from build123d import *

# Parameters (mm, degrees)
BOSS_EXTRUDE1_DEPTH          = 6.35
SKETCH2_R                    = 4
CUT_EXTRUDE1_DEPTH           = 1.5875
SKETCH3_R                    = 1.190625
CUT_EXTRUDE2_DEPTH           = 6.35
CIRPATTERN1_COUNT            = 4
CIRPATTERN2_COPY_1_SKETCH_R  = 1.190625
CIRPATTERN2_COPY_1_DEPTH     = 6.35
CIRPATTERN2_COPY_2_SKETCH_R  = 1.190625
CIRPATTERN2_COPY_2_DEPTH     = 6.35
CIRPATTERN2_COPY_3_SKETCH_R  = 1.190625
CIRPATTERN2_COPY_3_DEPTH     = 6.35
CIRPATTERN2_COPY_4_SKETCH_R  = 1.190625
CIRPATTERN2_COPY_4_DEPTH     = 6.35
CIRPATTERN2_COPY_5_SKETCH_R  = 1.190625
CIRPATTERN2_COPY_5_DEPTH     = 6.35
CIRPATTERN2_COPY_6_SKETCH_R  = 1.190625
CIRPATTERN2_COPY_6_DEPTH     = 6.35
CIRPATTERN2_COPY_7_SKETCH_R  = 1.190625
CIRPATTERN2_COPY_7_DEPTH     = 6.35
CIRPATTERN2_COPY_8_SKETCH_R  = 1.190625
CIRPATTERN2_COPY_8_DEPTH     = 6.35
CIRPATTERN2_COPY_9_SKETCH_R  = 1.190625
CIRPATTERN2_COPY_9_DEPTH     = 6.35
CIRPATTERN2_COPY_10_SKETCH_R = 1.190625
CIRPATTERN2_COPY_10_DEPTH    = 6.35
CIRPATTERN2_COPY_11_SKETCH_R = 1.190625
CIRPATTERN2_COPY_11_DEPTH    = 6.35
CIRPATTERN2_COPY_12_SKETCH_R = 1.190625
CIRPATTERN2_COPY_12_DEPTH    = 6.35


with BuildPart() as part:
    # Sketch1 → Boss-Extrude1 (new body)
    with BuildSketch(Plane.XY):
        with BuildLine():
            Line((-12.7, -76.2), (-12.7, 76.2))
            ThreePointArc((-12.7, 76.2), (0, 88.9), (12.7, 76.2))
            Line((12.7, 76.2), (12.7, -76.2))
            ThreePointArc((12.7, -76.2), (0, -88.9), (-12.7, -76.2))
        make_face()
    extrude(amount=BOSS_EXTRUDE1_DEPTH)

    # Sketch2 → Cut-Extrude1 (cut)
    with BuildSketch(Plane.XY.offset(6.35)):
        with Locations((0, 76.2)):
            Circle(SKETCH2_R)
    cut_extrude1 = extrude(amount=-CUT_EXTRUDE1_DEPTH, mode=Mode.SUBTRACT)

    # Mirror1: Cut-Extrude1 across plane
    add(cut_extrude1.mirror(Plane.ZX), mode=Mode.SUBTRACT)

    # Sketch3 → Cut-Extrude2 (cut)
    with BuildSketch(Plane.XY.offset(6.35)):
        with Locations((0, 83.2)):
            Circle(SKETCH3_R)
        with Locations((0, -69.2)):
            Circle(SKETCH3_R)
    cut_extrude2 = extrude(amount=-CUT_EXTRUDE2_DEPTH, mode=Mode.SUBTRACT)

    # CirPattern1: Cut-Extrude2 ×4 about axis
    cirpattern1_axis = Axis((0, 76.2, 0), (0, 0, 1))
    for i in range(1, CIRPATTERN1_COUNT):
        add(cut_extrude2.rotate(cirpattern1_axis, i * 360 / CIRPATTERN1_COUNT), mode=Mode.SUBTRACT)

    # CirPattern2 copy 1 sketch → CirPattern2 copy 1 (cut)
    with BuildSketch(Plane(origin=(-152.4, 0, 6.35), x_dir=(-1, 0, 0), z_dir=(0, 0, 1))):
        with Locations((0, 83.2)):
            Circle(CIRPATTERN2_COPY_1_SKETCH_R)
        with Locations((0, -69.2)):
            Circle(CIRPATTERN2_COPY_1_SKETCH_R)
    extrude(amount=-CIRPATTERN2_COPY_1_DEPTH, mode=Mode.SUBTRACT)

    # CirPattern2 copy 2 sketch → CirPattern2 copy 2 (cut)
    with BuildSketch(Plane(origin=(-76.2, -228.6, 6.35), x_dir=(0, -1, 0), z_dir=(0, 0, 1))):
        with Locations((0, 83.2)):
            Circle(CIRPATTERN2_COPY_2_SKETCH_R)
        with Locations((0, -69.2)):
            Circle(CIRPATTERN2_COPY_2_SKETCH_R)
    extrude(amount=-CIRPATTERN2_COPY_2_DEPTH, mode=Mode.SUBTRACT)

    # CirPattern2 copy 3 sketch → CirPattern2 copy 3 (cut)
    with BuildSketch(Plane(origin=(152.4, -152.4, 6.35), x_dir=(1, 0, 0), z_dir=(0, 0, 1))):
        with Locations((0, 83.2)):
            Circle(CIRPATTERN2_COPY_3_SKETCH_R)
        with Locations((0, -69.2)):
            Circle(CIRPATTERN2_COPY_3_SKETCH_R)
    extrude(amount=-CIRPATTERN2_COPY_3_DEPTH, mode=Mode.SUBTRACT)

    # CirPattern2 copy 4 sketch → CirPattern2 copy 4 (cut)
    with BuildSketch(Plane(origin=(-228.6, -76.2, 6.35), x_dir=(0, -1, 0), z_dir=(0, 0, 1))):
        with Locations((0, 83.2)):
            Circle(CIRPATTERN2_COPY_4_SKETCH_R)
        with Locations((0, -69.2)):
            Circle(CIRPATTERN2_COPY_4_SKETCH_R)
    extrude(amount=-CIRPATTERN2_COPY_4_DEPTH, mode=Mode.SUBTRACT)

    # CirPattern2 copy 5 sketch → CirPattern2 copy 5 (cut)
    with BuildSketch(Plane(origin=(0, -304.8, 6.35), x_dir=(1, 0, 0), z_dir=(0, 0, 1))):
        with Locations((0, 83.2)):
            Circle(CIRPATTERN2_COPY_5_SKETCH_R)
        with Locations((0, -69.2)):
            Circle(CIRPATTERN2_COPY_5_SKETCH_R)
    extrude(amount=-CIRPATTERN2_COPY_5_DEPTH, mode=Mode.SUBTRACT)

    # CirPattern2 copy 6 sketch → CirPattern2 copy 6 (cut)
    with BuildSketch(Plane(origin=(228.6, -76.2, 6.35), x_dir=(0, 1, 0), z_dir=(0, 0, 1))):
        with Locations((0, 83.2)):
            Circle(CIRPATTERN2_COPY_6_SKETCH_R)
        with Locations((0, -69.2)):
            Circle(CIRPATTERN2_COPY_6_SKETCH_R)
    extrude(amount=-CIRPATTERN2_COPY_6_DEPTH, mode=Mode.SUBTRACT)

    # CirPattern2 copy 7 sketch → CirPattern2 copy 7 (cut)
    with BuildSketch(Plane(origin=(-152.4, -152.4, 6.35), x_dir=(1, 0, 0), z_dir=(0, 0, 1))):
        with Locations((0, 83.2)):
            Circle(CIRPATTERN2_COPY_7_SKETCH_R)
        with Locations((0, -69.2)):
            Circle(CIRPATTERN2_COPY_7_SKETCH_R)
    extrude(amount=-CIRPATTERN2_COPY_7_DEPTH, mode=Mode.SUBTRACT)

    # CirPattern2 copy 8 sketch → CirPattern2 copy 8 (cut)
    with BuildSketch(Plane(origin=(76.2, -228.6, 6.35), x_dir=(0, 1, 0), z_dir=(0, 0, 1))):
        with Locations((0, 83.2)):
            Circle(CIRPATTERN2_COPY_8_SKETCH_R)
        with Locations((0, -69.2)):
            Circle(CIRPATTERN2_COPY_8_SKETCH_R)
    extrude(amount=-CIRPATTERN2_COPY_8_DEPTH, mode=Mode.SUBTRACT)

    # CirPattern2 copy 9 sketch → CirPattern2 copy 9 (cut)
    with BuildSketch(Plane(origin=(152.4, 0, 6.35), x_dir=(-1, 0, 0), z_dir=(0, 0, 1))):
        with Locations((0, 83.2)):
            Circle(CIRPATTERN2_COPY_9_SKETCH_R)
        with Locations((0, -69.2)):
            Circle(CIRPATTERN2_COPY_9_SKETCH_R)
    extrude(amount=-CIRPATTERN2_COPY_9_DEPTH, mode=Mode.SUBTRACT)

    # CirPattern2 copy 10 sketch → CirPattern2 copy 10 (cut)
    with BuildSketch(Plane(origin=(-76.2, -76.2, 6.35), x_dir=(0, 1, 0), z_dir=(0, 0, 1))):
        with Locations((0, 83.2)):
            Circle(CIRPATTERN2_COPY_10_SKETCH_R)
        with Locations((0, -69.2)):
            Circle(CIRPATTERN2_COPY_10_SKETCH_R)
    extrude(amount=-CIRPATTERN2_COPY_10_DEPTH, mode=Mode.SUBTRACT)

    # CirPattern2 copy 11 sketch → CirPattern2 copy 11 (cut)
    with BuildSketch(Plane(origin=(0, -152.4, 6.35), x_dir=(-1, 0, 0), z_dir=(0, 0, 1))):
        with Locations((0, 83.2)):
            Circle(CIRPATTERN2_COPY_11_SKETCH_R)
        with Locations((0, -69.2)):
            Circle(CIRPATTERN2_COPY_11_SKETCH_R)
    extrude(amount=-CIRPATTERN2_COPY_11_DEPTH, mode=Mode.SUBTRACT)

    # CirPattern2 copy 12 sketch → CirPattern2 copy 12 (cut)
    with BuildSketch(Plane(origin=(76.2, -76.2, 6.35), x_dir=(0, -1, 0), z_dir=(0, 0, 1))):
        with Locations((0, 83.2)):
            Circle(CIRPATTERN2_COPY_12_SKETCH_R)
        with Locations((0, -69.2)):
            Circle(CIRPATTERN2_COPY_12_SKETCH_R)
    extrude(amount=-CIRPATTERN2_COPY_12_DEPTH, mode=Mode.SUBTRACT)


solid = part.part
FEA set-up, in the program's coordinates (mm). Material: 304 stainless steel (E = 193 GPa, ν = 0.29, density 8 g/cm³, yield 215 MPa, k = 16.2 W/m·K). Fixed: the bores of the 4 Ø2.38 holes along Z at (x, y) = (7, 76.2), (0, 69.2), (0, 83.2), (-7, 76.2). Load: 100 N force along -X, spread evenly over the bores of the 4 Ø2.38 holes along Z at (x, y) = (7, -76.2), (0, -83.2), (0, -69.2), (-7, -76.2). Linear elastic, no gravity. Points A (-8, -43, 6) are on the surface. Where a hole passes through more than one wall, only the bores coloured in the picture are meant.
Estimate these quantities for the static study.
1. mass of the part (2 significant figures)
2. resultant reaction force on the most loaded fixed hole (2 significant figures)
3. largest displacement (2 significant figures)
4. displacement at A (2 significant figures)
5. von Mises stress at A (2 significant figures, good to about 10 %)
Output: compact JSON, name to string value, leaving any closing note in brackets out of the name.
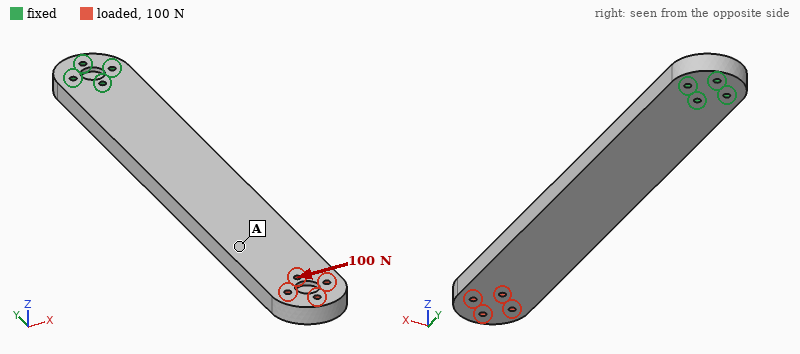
{"mass of the part": "220 g", "resultant reaction force on the most loaded fixed hole": "710 N", "largest displacement": "83 µm", "displacement at A": "51 µm", "von Mises stress at A": "3.1 MPa"}
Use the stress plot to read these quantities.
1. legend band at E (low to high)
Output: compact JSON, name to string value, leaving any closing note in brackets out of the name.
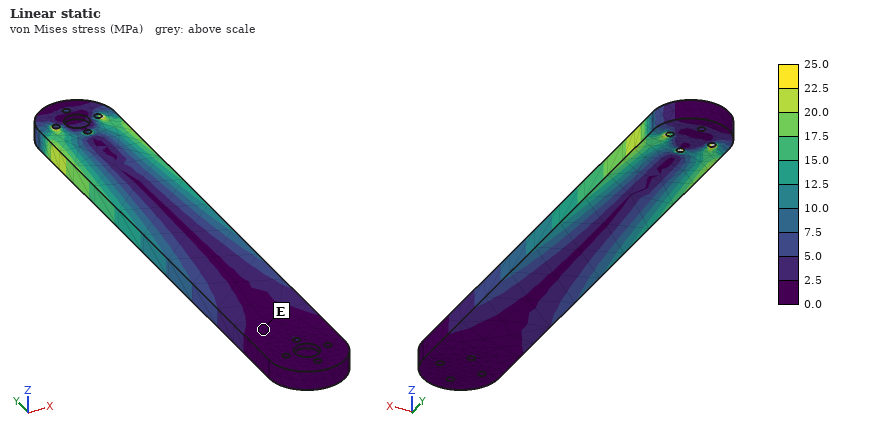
{"legend band at E": "0.0 to 2.5 MPa"}
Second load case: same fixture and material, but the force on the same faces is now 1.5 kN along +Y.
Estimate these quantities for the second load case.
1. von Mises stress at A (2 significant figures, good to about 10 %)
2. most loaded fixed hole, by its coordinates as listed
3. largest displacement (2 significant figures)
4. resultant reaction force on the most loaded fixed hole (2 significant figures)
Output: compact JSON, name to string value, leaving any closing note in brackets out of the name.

{"von Mises stress at A": "9.3 MPa", "most loaded fixed hole, by its coordinates as listed": "(0, 69.2)", "largest displacement": "7.7 µm", "resultant reaction force on the most loaded fixed hole": "690 N"}
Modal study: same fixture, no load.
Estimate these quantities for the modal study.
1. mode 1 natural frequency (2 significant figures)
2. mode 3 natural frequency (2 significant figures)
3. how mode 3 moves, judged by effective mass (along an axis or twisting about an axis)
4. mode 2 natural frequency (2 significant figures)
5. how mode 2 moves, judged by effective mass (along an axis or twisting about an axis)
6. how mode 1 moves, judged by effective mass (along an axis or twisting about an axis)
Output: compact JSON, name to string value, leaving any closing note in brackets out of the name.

{"mode 1 natural frequency": "210 Hz", "mode 3 natural frequency": "1300 Hz", "how mode 3 moves, judged by effective mass": "along Z", "mode 2 natural frequency": "750 Hz", "how mode 2 moves, judged by effective mass": "along X", "how mode 1 moves, judged by effective mass": "along Z"}
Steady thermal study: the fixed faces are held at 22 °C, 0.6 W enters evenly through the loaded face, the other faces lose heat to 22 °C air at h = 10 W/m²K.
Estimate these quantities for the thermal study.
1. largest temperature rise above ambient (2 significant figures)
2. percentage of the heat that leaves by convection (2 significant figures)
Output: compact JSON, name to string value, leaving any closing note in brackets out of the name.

{"largest temperature rise above ambient": "13 K", "percentage of the heat that leaves by convection": "83 %"}
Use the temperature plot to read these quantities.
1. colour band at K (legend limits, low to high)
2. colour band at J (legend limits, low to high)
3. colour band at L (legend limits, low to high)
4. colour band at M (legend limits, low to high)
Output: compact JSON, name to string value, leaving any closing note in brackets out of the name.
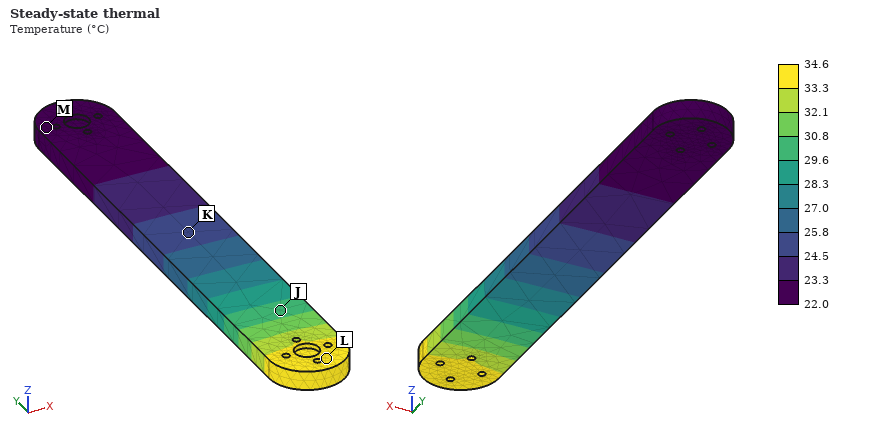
{"colour band at K": "24.5 to 25.8 °C", "colour band at J": "29.6 to 30.8 °C", "colour band at L": "33.3 to 34.6 °C", "colour band at M": "22.0 to 23.3 °C"}
